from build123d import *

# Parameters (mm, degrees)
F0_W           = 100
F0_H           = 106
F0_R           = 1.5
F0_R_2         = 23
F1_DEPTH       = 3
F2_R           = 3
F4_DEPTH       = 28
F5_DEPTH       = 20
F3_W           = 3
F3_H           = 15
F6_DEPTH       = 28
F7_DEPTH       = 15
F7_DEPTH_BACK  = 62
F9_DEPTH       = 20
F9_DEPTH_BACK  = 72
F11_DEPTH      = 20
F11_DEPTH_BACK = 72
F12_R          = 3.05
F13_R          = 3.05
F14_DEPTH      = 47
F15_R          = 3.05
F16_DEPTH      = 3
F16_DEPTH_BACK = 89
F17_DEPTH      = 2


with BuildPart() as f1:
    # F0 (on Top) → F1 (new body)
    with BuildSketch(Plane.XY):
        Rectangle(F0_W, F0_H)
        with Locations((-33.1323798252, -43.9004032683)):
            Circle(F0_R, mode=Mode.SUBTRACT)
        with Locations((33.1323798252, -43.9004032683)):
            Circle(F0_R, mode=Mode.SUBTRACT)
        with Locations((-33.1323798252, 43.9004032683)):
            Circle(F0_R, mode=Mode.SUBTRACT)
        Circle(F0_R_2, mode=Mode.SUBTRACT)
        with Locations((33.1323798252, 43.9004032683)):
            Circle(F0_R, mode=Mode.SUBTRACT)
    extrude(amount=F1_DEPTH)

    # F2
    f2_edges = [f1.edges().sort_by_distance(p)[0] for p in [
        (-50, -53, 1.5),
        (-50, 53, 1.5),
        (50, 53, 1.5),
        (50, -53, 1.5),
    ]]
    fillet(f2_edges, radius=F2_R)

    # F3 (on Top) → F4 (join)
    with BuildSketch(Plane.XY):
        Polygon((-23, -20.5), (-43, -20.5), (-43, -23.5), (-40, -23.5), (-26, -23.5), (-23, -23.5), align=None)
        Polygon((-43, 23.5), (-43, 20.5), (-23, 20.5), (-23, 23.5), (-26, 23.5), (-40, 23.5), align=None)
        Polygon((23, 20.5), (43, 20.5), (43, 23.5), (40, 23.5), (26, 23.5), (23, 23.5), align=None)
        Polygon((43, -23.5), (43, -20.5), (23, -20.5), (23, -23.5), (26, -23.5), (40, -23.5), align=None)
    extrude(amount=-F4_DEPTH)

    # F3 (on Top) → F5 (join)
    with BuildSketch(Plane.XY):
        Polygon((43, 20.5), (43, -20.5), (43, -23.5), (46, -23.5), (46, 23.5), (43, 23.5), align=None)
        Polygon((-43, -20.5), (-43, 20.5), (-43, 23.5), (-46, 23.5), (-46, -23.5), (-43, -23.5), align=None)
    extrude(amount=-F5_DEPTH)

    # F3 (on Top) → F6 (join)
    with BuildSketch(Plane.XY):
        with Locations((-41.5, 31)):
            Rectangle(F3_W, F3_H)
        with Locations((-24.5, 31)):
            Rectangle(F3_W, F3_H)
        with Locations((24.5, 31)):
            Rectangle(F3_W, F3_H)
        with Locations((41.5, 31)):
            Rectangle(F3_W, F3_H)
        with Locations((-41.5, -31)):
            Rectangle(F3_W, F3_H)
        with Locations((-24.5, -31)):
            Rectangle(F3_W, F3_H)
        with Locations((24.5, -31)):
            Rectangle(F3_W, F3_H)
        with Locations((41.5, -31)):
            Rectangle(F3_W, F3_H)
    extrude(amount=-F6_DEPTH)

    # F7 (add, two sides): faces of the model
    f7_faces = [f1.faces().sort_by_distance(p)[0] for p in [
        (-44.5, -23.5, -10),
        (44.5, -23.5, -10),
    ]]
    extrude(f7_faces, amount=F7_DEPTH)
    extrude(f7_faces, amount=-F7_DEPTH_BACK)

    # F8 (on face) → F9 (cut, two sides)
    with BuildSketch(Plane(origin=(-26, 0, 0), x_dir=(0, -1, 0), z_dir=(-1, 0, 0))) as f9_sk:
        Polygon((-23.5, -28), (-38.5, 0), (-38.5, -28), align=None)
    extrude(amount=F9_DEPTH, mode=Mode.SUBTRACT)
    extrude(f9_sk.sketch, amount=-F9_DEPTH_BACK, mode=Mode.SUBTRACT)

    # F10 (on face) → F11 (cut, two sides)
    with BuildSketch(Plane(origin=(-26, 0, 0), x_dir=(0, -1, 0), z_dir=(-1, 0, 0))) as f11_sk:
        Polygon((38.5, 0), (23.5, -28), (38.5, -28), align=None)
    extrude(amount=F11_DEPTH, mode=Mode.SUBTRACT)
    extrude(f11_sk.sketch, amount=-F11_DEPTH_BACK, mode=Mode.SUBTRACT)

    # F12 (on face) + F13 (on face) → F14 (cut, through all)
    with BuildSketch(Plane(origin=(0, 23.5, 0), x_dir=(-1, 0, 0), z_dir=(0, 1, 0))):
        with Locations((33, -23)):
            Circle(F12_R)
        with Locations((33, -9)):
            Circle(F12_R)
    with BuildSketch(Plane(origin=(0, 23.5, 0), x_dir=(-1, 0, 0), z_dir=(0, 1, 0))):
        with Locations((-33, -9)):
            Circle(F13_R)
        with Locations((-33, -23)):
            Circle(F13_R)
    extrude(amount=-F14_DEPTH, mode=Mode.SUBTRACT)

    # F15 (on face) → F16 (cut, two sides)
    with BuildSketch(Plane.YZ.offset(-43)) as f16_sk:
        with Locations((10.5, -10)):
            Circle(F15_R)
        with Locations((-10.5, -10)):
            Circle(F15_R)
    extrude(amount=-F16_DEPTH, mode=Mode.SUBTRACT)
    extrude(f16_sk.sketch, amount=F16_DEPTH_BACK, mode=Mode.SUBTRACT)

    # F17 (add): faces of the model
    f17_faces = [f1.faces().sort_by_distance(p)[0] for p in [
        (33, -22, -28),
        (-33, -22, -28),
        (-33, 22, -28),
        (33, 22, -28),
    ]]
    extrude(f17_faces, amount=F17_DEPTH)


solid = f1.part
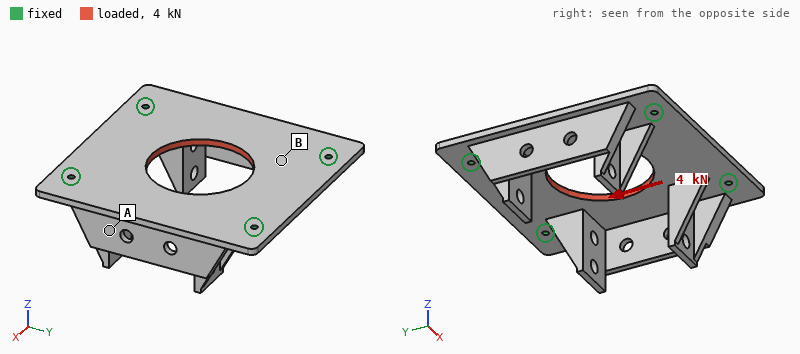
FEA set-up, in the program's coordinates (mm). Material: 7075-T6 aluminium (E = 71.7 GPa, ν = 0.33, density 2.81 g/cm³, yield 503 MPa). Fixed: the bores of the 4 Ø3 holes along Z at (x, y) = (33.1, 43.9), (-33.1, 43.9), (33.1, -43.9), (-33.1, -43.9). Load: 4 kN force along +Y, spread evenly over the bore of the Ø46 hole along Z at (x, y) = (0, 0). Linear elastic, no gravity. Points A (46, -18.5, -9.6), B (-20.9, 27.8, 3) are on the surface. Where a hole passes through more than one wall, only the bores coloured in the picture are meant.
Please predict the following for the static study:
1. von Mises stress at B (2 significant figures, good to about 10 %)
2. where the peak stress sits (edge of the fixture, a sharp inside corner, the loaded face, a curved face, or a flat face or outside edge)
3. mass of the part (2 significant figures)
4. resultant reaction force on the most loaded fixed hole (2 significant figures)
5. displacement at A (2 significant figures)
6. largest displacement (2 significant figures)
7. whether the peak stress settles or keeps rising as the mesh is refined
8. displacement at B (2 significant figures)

12 MPa
edge of the fixture
130 g
1.0 kN
3.4 µm
11 µm
keeps rising
6.3 µm
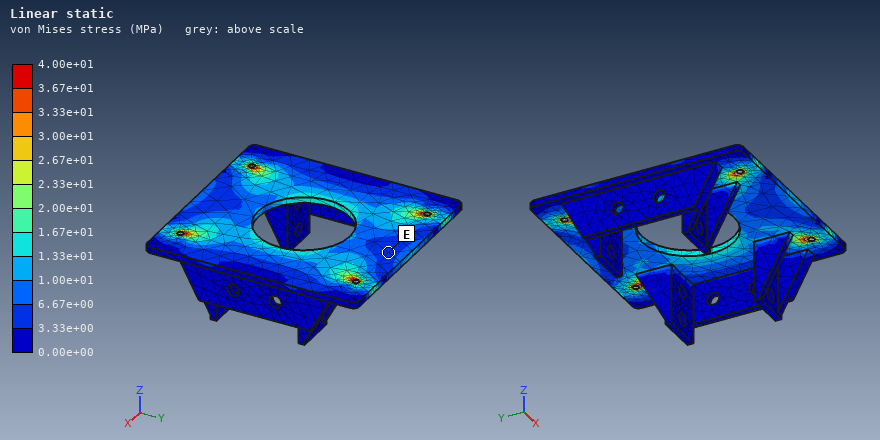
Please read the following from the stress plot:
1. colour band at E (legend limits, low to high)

3.33e+00 to 6.67e+00 MPa
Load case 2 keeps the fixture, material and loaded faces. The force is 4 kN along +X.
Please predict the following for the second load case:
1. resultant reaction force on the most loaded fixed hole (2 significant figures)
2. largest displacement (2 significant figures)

1.0 kN
18 µm
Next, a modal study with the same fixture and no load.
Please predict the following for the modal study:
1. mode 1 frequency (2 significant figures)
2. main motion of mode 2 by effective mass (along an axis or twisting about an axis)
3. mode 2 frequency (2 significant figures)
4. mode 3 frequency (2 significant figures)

1800 Hz
along X
2600 Hz
2700 Hz
